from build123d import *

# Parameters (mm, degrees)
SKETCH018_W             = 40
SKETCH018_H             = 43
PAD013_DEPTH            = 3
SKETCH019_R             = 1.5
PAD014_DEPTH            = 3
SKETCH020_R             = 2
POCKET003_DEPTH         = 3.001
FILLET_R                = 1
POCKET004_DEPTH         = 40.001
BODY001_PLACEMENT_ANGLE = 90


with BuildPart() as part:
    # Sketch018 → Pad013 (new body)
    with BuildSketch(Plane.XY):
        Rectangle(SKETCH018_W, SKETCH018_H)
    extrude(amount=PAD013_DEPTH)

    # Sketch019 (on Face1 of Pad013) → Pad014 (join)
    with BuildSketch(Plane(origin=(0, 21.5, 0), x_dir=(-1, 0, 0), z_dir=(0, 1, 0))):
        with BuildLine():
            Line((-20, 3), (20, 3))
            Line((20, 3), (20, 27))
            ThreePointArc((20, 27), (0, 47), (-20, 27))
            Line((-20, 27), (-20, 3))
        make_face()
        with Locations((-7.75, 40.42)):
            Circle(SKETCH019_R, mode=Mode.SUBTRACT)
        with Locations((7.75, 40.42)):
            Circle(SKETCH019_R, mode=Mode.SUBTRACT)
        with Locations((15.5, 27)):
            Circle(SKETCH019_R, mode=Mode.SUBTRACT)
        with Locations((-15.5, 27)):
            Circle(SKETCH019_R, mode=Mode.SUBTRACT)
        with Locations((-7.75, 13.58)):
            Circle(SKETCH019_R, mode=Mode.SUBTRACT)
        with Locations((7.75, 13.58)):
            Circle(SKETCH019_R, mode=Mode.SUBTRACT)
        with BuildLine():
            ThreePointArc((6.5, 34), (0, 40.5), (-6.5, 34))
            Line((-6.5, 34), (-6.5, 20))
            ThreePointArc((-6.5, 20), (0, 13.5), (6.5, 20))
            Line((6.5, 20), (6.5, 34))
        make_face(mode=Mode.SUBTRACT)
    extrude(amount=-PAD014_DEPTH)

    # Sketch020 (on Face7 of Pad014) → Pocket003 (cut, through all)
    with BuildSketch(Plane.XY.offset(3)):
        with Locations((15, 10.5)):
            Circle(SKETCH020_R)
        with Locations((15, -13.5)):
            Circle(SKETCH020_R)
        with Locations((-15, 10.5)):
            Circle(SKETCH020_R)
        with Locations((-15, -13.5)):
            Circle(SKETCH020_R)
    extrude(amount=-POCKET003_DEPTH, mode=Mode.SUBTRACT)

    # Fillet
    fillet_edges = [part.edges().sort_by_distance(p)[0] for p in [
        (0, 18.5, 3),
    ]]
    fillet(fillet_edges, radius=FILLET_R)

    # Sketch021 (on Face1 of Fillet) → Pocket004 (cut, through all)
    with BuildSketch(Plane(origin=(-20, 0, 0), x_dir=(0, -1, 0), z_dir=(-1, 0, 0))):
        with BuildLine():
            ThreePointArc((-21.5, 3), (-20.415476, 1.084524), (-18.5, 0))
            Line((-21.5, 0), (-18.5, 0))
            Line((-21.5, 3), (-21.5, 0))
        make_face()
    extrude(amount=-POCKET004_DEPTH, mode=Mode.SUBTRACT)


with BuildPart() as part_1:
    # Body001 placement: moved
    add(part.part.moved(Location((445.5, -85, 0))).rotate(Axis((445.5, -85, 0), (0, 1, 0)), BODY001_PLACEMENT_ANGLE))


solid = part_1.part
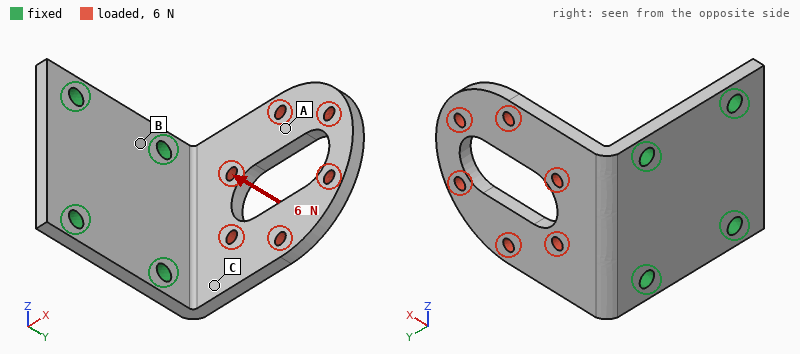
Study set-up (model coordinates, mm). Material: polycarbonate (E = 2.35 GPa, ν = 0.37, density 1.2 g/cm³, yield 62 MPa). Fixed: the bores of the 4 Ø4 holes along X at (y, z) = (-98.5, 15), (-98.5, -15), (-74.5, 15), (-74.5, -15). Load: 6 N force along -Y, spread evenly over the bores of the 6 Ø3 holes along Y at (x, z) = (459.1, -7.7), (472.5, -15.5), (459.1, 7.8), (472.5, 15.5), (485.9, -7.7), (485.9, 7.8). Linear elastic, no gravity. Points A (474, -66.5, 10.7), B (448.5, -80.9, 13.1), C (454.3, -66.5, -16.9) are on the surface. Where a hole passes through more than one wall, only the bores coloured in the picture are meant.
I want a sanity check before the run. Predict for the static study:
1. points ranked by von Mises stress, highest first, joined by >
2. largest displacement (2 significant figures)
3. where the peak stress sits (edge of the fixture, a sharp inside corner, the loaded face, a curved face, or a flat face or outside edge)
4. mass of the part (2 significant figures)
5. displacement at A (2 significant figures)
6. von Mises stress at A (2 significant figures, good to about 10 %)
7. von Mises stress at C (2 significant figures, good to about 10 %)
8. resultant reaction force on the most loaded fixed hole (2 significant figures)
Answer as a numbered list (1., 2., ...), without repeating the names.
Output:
1. C > A > B
2. 0.69 mm
3. a flat face or outside edge
4. 10 g
5. 0.34 mm
6. 0.77 MPa
7. 1.9 MPa
8. 2.2 N
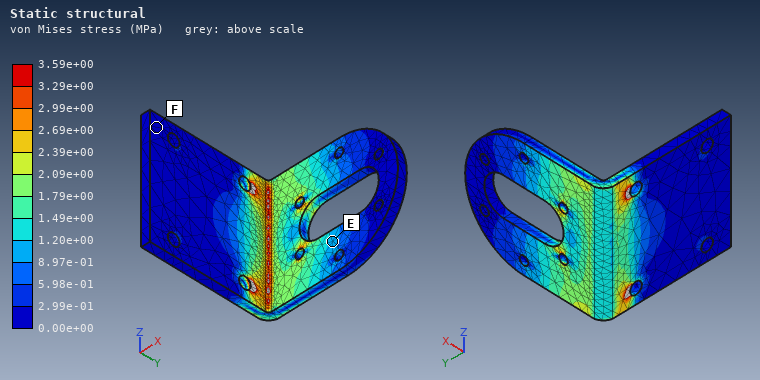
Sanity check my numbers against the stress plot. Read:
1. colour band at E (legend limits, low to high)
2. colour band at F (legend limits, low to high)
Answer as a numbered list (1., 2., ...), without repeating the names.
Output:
1. 8.97e-01 to 1.20e+00 MPa
2. 0.00e+00 to 2.99e-01 MPa
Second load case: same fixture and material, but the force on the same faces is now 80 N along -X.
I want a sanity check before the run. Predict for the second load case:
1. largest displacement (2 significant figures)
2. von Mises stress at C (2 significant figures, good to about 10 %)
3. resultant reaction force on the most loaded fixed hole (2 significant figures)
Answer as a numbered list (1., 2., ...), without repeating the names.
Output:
1. 0.73 mm
2. 1.5 MPa
3. 43 N
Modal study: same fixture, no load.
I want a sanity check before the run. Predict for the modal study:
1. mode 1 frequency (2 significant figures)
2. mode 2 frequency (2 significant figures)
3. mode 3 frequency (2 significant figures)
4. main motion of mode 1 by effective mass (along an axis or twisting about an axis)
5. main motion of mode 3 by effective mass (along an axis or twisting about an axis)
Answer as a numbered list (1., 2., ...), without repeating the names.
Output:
1. 330 Hz
2. 840 Hz
3. 1300 Hz
4. along Y
5. along Z
